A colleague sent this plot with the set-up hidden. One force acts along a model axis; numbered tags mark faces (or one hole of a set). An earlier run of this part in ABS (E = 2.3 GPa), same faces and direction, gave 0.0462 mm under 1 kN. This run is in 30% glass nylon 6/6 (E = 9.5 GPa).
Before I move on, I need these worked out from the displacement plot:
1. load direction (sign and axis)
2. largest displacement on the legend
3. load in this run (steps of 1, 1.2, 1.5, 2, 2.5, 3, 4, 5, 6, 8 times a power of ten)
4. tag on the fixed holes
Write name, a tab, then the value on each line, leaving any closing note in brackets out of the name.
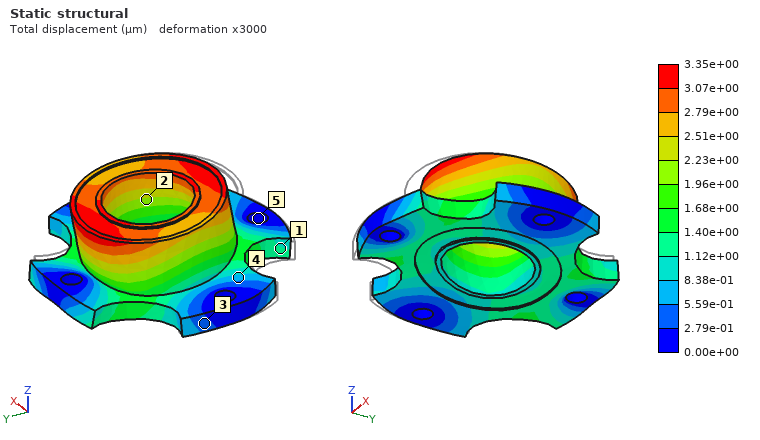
load direction	+Y
largest displacement on the legend	3.35e+00 µm
load in this run	300 N
tag on the fixed holes	5
